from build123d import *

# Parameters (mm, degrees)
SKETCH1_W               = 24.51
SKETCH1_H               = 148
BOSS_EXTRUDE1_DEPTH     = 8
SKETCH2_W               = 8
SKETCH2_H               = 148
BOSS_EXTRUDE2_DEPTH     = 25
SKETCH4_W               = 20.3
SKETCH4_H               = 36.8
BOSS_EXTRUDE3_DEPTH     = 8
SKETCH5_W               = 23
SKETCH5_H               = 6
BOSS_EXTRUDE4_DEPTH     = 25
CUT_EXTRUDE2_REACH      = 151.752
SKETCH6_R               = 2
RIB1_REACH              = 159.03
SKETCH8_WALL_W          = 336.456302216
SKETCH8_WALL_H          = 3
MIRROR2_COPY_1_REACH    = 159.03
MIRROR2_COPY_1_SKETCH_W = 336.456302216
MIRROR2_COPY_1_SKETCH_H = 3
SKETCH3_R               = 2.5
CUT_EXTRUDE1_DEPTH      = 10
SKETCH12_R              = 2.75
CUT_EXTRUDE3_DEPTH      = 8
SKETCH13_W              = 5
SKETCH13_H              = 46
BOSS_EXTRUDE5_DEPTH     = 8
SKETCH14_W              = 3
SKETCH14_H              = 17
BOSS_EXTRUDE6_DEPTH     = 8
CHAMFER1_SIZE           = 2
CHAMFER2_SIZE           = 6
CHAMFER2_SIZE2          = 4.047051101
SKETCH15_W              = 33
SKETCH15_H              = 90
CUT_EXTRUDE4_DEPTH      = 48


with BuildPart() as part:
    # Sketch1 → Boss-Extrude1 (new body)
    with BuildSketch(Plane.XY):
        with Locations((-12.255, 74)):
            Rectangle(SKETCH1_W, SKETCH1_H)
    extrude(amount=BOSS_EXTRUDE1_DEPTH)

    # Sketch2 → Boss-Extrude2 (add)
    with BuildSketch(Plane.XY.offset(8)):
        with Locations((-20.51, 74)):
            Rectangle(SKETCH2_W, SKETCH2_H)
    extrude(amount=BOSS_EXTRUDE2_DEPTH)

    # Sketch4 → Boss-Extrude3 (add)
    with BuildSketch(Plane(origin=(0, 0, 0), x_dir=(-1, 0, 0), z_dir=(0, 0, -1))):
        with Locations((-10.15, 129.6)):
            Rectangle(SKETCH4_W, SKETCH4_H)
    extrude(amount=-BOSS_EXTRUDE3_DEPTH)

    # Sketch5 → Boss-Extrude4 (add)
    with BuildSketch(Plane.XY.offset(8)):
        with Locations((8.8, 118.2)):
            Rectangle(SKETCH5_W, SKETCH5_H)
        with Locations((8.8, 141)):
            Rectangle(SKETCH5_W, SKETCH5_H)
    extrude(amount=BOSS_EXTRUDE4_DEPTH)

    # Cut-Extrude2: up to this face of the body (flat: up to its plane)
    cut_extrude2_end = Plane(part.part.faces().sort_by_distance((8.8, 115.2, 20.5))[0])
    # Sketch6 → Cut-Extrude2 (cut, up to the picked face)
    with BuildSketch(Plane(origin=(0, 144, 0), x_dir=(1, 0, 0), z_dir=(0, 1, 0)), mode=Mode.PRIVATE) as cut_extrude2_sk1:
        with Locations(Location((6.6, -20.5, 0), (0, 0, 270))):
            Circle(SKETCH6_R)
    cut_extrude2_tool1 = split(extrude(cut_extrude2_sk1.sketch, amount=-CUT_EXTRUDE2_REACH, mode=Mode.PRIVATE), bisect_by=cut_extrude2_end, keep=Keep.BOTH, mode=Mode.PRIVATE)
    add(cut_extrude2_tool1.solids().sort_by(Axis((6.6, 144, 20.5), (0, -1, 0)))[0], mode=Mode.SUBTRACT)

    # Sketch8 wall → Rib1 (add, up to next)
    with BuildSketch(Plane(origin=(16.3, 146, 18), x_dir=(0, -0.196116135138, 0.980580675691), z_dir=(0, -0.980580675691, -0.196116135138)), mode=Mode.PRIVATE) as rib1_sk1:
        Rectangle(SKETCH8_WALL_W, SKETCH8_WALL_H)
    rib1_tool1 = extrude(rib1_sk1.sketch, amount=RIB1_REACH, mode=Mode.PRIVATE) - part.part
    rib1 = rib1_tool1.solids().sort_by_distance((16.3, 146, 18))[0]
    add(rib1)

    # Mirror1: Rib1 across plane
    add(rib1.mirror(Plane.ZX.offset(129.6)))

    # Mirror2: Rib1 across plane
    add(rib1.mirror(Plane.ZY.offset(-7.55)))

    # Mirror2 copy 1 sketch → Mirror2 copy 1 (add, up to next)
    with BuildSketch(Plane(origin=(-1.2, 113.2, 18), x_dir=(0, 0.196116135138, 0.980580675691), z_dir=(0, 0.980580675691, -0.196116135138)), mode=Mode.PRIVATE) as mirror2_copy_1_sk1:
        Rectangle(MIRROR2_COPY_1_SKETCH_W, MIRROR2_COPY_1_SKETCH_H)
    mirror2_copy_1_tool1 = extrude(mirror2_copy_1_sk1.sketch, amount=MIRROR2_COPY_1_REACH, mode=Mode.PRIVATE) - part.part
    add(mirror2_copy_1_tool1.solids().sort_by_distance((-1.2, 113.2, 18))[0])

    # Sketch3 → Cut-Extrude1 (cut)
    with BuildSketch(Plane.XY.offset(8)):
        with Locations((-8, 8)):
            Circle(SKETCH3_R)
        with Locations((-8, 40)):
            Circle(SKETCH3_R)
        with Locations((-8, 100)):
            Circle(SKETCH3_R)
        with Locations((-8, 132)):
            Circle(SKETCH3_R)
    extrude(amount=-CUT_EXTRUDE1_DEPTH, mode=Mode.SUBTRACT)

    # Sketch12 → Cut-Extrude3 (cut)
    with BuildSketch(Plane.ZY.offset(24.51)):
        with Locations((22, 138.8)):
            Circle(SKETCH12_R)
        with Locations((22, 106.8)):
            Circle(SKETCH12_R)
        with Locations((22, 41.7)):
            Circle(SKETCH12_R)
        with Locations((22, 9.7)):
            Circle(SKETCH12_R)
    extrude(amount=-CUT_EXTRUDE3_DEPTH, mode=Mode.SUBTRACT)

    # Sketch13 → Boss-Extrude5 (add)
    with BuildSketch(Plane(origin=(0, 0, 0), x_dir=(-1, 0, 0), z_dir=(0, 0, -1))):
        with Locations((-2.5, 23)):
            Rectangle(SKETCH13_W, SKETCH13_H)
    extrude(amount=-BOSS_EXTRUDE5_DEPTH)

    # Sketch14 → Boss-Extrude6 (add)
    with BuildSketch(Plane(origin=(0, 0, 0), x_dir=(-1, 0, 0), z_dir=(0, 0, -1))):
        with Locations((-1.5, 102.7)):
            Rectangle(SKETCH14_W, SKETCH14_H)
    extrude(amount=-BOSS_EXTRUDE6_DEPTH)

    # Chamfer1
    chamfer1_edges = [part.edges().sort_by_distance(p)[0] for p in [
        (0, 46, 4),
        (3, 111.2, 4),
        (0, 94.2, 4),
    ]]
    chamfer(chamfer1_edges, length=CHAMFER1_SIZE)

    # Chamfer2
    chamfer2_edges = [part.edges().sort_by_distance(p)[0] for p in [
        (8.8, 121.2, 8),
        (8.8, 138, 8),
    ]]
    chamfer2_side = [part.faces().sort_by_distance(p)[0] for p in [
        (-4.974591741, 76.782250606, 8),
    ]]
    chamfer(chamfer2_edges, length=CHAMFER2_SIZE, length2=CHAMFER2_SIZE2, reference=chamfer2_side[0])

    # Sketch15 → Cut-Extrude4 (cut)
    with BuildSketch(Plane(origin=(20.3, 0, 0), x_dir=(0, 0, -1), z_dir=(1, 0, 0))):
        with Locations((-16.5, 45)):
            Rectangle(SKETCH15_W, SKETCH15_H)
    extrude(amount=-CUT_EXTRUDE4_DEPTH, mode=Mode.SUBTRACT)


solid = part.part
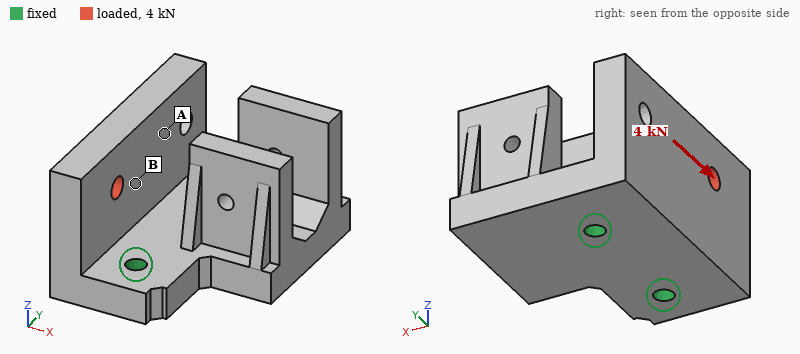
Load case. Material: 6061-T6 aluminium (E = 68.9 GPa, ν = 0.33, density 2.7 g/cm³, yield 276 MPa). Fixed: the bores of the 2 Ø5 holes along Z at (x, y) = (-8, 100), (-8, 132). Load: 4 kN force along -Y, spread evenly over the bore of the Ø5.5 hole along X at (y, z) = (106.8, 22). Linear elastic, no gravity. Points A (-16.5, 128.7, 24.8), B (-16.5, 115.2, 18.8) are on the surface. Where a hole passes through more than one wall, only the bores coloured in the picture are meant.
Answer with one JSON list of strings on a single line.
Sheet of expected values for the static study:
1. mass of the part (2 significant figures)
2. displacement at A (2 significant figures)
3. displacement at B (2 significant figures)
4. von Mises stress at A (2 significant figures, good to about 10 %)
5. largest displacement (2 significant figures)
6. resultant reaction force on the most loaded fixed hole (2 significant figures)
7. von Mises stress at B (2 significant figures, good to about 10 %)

["99 g", "33 µm", "25 µm", "17 MPa", "52 µm", "3.1 kN", "33 MPa"]
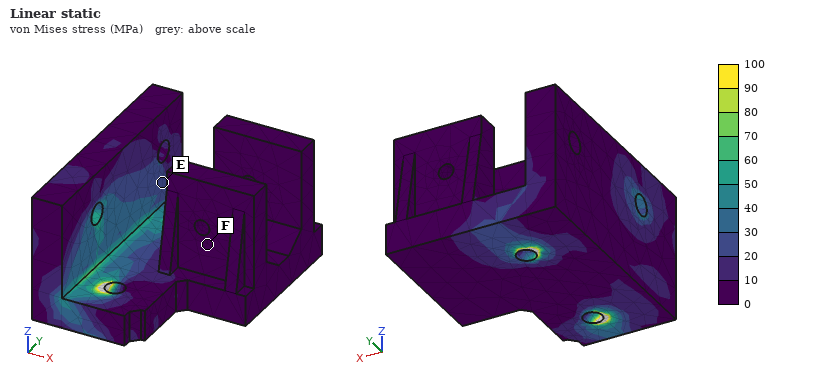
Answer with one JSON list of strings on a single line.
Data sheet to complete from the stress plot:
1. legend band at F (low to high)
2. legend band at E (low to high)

["0 to 10 MPa", "20 to 30 MPa"]
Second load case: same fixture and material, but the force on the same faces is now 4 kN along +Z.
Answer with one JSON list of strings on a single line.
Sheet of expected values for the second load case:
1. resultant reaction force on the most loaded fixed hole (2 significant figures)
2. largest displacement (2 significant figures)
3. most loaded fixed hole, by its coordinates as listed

["3.0 kN", "99 µm", "(-8, 100)"]
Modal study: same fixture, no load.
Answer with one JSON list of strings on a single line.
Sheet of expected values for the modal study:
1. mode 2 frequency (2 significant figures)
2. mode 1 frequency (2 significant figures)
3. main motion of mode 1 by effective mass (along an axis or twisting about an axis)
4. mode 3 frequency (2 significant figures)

["4900 Hz", "3800 Hz", "along X", "5800 Hz"]
